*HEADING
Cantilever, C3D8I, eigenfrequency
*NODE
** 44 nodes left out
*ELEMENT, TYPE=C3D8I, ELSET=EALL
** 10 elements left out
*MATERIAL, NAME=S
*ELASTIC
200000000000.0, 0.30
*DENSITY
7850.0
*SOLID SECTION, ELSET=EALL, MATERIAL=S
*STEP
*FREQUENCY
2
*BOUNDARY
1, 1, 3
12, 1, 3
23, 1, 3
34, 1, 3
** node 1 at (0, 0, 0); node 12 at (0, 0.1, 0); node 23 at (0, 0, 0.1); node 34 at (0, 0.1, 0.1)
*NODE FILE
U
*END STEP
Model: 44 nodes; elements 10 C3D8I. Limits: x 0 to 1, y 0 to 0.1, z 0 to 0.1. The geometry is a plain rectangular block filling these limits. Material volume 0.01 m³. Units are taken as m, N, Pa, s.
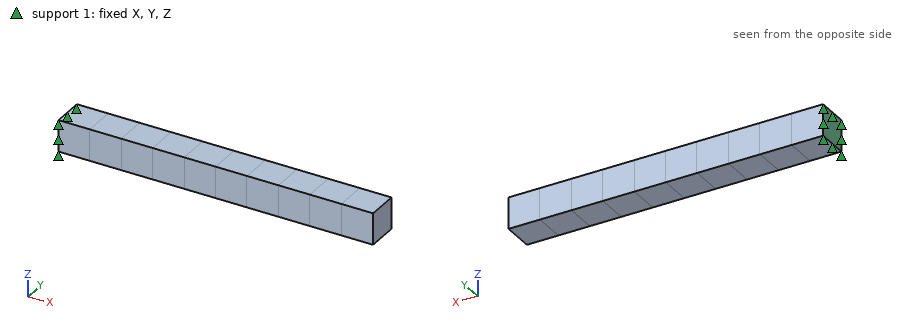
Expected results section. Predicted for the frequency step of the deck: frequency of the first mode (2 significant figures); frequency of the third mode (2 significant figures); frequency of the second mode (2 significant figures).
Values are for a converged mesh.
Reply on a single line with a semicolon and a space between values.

82 Hz; 490 Hz; 82 Hz
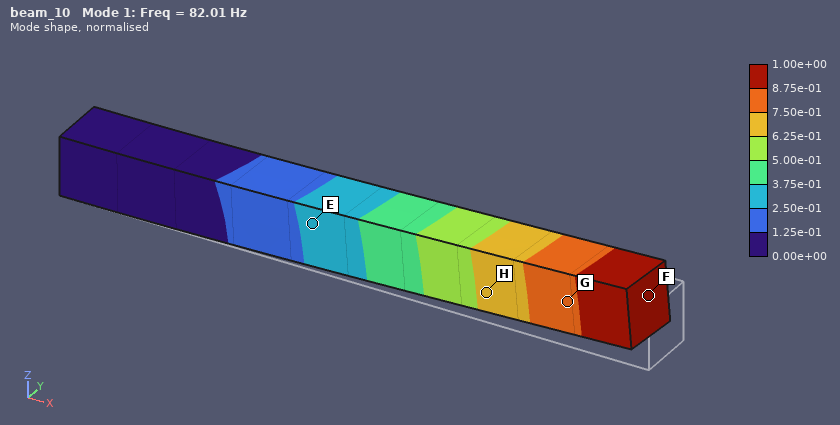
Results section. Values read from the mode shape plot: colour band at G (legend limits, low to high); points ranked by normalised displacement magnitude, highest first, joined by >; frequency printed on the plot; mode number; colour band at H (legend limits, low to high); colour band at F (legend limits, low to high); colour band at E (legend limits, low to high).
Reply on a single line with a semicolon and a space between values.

7.50e-01 to 8.75e-01; F > G > H > E; 82.01 Hz; 1; 6.25e-01 to 7.50e-01; 8.75e-01 to 1.00e+00; 2.50e-01 to 3.75e-01
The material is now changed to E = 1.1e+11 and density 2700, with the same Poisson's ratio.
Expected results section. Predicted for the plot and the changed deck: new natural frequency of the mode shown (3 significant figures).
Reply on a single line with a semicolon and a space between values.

104 Hz
